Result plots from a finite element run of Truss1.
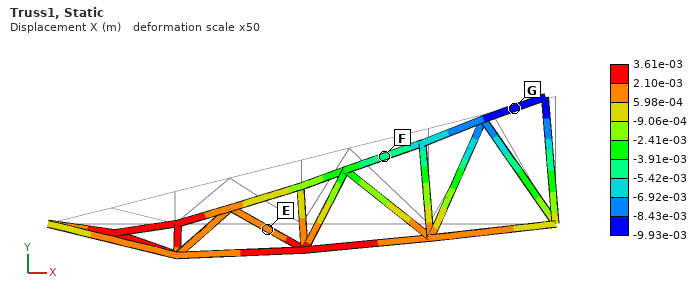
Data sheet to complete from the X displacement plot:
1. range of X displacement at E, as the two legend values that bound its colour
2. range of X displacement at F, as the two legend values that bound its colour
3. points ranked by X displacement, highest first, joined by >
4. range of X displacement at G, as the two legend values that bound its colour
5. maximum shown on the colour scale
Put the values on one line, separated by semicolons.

5.98e-04 to 2.10e-03 m; -5.42e-03 to -3.91e-03 m; E > F > G; -9.93e-03 to -8.43e-03 m; 3.61e-03 m
